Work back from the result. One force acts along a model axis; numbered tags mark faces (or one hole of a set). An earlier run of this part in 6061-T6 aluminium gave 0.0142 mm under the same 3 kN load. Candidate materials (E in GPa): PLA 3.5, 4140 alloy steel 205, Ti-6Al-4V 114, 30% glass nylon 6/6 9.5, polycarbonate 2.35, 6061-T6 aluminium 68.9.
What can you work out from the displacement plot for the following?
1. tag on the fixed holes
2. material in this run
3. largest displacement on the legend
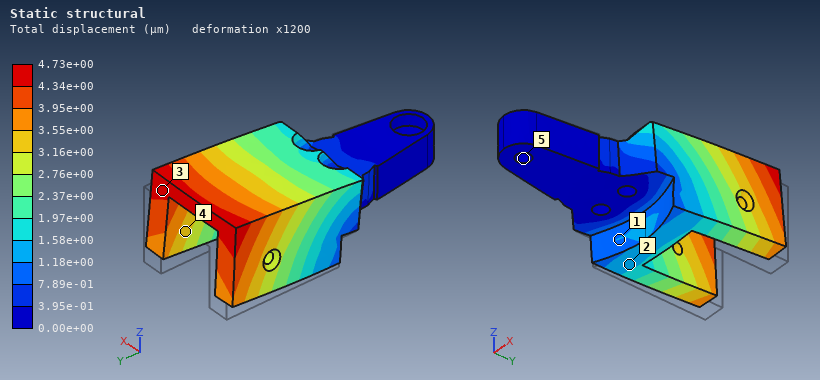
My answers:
5
4140 alloy steel
4.73e+00 µm
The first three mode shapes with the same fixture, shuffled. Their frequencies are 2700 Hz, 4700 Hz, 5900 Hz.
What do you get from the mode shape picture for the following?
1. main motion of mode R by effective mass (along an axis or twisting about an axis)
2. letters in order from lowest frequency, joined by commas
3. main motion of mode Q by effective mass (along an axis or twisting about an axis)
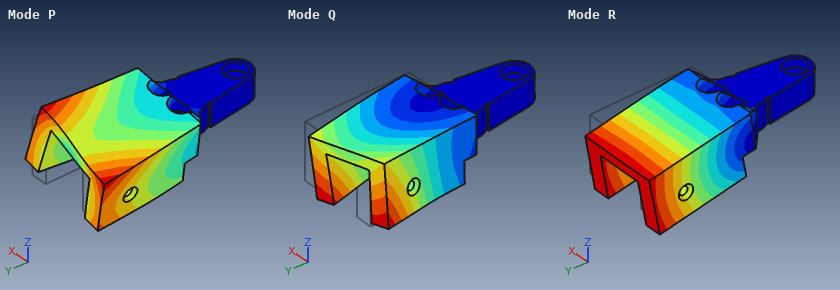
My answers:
along Z
R, Q, P
along X
